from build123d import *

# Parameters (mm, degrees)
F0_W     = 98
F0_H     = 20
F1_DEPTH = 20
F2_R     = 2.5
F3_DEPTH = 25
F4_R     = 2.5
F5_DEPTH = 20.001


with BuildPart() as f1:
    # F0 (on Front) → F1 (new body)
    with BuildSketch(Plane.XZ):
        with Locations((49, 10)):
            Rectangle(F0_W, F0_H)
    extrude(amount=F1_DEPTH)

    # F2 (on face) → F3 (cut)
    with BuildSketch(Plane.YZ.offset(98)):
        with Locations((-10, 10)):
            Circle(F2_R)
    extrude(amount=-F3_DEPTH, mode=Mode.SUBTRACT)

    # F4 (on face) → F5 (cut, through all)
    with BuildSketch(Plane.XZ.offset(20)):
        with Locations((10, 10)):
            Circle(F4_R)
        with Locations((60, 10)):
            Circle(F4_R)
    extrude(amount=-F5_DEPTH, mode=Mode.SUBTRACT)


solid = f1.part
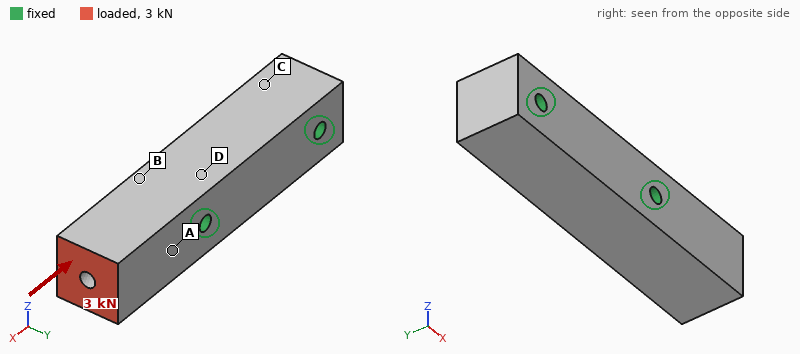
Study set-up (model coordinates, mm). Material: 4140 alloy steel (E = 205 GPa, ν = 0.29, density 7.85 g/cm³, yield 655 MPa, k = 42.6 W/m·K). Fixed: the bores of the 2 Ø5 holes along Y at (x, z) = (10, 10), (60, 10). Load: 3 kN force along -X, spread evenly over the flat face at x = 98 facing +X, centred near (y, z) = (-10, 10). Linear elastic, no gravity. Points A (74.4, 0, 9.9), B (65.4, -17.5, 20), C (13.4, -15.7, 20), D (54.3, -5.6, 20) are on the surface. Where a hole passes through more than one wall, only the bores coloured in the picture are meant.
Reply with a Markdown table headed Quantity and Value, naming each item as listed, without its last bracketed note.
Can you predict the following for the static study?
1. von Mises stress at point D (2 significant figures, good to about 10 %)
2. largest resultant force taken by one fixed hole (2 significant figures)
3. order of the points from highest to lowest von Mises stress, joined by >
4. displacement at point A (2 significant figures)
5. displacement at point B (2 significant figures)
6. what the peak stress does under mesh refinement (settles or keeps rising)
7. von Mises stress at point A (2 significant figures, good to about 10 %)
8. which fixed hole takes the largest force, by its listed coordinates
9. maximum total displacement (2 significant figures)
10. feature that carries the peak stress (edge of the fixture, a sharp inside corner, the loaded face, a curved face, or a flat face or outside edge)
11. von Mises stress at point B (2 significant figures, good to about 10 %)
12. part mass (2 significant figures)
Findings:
| Quantity | Value |
|---|---|
| von Mises stress at point D | 2.9 MPa |
| largest resultant force taken by one fixed hole | 2.8 kN |
| order of the points from highest to lowest von Mises stress, joined by > | A > B > D > C |
| displacement at point A | 0.63 µm |
| displacement at point B | 0.39 µm |
| what the peak stress does under mesh refinement | keeps rising |
| von Mises stress at point A | 8.4 MPa |
| which fixed hole takes the largest force, by its listed coordinates | (60, 10) |
| maximum total displacement | 1.5 µm |
| feature that carries the peak stress | edge of the fixture |
| von Mises stress at point B | 4.5 MPa |
| part mass | 300 g |
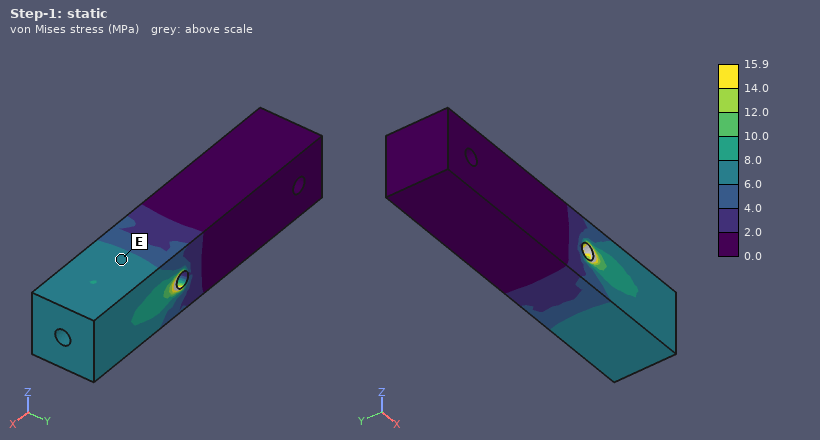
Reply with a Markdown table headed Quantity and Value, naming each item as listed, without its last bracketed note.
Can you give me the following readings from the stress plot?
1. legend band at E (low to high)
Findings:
| Quantity | Value |
|---|---|
| legend band at E | 6.0 to 8.0 MPa |
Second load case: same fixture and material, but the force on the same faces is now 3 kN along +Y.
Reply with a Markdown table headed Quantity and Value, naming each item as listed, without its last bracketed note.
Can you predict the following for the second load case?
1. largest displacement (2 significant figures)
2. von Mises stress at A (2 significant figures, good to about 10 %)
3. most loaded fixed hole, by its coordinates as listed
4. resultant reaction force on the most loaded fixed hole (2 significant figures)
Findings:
| Quantity | Value |
|---|---|
| largest displacement | 28 µm |
| von Mises stress at A | 57 MPa |
| most loaded fixed hole, by its coordinates as listed | (60, 10) |
| resultant reaction force on the most loaded fixed hole | 3.4 kN |
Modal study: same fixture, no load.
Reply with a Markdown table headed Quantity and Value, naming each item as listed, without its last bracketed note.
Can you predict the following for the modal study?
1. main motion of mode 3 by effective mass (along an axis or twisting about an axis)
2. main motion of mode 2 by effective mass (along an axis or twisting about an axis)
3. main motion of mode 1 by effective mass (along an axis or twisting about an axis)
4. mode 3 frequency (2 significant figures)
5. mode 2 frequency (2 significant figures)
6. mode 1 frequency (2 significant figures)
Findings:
| Quantity | Value |
|---|---|
| main motion of mode 3 by effective mass | twisting about X |
| main motion of mode 2 by effective mass | along Y |
| main motion of mode 1 by effective mass | along Z |
| mode 3 frequency | 19 kHz |
| mode 2 frequency | 9400 Hz |
| mode 1 frequency | 7500 Hz |
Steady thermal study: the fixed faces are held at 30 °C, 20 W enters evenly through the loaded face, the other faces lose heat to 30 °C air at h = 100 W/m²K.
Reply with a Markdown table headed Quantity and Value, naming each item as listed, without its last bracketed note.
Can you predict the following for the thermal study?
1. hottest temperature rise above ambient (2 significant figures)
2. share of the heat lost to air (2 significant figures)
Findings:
| Quantity | Value |
|---|---|
| hottest temperature rise above ambient | 37 K |
| share of the heat lost to air | 32 % |
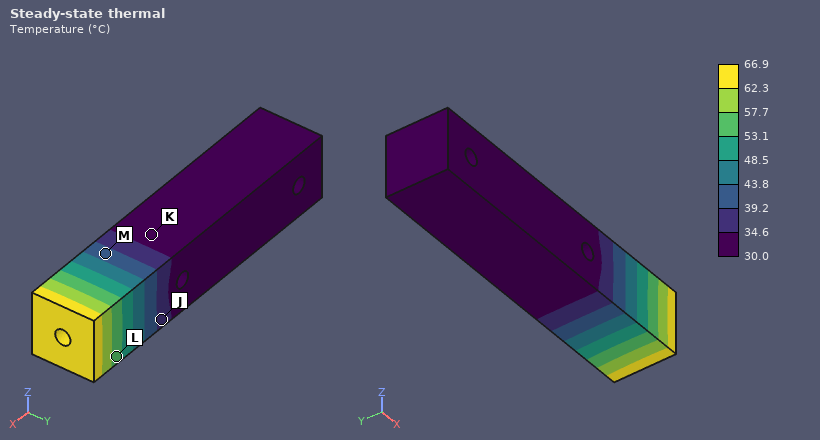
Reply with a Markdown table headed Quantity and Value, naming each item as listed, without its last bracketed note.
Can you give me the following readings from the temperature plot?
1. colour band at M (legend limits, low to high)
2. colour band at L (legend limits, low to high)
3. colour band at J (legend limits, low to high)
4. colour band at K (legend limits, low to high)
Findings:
| Quantity | Value |
|---|---|
| colour band at M | 39.2 to 43.8 °C |
| colour band at L | 53.1 to 57.7 °C |
| colour band at J | 34.6 to 39.2 °C |
| colour band at K | 30.0 to 34.6 °C |
